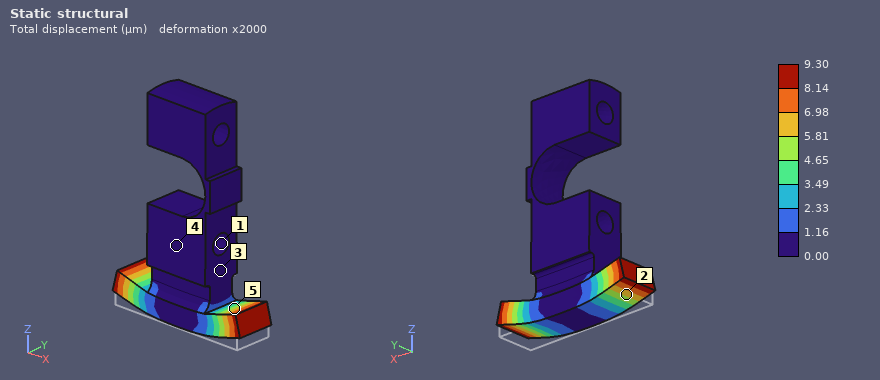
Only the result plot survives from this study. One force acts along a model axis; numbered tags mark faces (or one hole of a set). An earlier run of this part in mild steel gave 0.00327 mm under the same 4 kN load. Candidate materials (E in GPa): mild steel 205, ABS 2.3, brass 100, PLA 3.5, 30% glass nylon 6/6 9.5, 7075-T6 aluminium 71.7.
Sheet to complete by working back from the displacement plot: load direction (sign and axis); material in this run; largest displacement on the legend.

+Z
7075-T6 aluminium
9.30 µm
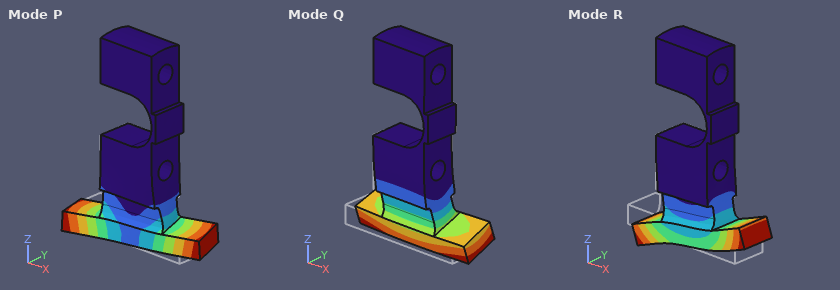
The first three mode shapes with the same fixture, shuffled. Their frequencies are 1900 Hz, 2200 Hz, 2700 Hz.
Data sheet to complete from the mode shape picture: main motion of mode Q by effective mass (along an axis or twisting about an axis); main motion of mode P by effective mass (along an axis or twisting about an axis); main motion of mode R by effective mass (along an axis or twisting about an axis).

along Y
twisting about Z
along X
